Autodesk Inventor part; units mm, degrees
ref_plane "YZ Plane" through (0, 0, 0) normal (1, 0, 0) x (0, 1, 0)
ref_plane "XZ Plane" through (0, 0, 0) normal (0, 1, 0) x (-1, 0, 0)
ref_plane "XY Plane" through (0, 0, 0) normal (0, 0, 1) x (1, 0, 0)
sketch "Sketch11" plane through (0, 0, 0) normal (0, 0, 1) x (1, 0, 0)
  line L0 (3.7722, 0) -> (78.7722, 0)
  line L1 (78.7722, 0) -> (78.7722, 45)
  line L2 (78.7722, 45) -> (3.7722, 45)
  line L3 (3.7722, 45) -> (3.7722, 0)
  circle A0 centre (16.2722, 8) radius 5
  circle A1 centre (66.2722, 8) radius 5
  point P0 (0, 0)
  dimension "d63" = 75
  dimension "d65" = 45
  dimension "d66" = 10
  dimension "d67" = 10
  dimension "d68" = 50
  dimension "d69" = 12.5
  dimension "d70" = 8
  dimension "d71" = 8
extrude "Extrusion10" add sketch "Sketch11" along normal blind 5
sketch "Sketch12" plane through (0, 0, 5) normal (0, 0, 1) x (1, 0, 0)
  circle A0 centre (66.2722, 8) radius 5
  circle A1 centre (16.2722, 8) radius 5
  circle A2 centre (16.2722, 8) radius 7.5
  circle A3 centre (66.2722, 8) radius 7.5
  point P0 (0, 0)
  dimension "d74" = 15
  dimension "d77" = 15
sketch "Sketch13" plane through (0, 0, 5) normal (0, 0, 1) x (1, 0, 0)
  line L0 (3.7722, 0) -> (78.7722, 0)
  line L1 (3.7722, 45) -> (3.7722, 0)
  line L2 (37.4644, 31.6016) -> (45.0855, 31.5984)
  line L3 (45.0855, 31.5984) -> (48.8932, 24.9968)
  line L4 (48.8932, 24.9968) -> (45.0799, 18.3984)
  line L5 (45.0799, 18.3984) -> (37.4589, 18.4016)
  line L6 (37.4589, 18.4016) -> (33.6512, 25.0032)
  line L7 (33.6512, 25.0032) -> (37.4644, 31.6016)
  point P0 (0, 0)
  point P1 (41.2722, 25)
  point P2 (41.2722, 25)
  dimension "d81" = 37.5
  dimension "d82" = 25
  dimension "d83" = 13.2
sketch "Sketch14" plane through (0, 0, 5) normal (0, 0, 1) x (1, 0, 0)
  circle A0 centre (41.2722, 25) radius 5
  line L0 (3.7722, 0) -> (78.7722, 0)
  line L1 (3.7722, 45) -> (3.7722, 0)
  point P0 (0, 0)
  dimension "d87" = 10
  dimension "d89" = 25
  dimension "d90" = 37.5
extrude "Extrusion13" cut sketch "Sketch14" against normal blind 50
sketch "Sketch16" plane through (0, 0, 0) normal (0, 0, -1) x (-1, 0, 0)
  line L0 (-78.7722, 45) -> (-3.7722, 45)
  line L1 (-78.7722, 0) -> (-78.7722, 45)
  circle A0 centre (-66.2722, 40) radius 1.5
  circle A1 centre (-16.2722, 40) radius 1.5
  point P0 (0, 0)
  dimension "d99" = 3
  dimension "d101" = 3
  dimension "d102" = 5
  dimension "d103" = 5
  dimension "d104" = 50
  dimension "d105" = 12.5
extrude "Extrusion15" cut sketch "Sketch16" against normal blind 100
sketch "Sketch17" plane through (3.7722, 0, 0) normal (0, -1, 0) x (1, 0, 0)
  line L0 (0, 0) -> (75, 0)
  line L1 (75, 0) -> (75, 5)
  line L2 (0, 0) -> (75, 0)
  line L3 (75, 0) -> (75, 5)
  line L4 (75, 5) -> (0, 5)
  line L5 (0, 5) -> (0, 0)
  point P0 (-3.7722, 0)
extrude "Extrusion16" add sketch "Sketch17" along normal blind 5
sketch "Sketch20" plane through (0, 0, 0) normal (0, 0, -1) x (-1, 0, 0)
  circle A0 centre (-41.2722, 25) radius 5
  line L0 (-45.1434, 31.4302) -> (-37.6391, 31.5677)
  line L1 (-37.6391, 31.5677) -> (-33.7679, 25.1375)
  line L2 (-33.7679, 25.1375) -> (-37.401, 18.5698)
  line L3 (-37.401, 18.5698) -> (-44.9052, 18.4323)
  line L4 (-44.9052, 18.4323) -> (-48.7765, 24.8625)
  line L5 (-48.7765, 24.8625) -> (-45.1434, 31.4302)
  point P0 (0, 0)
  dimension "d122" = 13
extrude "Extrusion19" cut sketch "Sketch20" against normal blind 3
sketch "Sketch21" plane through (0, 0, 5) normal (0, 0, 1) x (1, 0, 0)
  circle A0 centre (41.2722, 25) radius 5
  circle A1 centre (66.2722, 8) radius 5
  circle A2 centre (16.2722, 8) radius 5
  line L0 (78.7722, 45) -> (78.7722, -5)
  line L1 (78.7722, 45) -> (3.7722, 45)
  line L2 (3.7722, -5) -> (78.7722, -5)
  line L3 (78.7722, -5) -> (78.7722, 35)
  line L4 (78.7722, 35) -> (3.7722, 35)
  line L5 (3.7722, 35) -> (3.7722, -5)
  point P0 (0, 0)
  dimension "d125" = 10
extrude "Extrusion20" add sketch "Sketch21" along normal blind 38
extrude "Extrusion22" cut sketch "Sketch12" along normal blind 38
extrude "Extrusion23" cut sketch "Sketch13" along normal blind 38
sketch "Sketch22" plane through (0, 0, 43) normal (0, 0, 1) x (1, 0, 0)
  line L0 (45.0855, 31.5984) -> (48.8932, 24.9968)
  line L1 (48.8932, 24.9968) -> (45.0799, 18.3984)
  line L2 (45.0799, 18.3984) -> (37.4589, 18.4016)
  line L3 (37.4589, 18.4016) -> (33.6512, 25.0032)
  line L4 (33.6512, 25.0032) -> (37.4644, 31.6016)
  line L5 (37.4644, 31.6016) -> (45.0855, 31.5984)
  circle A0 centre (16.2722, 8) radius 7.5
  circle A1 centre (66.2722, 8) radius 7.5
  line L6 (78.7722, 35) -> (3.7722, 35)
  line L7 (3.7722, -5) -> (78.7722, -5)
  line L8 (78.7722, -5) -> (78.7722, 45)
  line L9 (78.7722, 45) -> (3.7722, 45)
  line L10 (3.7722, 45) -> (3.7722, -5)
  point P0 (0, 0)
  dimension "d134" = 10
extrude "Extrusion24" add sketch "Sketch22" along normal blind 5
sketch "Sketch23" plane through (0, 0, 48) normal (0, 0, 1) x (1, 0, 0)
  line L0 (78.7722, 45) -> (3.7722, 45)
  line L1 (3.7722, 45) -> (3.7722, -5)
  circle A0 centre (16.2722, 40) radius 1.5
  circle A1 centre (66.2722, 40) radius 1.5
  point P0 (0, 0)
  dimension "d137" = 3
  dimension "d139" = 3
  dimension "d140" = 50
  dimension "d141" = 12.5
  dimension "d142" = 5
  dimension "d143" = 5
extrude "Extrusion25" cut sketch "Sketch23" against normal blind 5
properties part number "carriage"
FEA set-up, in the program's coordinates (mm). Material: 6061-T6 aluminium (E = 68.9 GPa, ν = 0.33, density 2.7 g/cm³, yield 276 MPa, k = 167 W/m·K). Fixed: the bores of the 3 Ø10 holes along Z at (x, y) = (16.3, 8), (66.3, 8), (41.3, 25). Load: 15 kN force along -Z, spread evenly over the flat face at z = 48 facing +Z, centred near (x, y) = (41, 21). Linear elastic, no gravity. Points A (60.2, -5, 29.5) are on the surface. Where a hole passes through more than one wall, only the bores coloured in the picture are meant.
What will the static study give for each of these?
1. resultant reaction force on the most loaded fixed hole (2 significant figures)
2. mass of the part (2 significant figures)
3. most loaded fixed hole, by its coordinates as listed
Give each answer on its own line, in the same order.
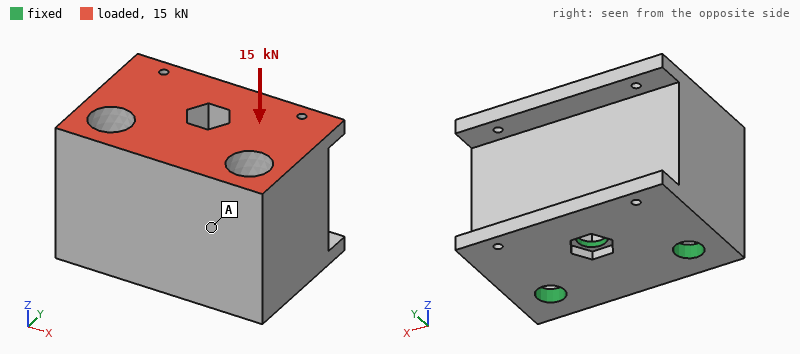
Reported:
8.3 kN
350 g
(41.3, 25)
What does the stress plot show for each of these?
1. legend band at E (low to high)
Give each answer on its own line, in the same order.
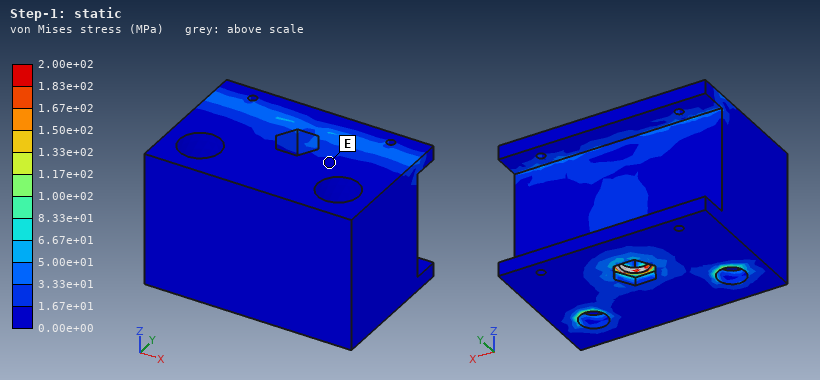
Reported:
0.00e+00 to 1.67e+01 MPa
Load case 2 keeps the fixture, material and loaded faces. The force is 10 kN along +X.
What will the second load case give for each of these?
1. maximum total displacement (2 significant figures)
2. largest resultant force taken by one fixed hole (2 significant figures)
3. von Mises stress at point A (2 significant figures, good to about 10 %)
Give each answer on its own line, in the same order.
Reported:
52 µm
9.2 kN
12 MPa
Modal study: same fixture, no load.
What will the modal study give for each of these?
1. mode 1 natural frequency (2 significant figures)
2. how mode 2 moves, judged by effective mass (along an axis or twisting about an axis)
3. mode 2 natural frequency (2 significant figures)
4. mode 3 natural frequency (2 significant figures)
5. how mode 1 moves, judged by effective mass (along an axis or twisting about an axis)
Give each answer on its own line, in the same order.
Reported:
3300 Hz
along X
6500 Hz
8900 Hz
along Y
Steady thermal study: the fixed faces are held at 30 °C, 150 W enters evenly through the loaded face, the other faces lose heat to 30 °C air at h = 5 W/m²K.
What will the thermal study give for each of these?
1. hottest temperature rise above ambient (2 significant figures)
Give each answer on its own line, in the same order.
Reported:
31 K
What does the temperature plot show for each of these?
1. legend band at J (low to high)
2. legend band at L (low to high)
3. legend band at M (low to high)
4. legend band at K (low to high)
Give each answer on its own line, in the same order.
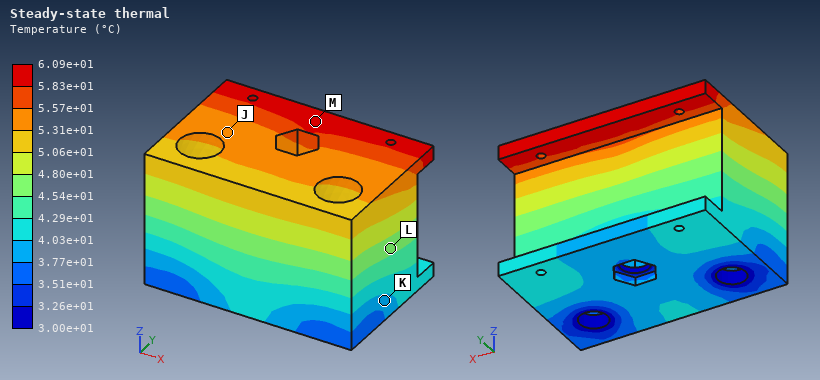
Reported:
5.31e+01 to 5.57e+01 °C
4.54e+01 to 4.80e+01 °C
5.83e+01 to 6.09e+01 °C
3.77e+01 to 4.03e+01 °C
